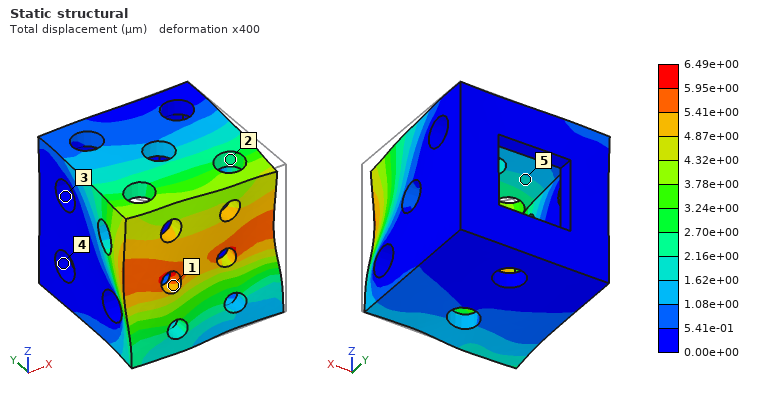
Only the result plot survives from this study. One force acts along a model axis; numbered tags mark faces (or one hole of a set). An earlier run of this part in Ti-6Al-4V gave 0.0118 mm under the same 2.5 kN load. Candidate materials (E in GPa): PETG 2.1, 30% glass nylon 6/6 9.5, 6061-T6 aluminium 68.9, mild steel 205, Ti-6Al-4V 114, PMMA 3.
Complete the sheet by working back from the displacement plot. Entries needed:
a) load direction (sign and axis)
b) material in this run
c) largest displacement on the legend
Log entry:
-X
mild steel
6.49e+00 µm
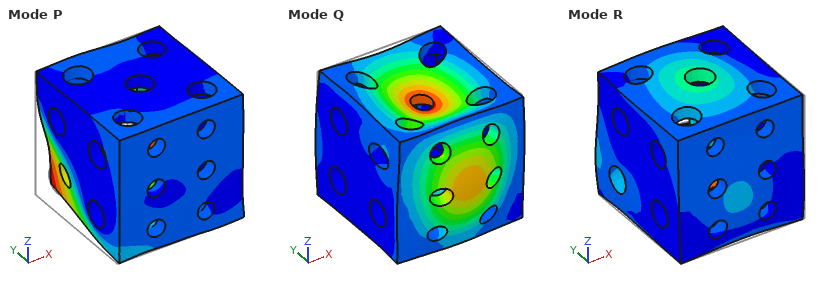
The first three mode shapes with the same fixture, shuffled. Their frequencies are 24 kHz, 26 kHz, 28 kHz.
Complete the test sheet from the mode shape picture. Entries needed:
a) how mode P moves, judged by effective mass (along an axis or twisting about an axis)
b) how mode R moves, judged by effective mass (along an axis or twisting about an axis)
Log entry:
along X
along Z
